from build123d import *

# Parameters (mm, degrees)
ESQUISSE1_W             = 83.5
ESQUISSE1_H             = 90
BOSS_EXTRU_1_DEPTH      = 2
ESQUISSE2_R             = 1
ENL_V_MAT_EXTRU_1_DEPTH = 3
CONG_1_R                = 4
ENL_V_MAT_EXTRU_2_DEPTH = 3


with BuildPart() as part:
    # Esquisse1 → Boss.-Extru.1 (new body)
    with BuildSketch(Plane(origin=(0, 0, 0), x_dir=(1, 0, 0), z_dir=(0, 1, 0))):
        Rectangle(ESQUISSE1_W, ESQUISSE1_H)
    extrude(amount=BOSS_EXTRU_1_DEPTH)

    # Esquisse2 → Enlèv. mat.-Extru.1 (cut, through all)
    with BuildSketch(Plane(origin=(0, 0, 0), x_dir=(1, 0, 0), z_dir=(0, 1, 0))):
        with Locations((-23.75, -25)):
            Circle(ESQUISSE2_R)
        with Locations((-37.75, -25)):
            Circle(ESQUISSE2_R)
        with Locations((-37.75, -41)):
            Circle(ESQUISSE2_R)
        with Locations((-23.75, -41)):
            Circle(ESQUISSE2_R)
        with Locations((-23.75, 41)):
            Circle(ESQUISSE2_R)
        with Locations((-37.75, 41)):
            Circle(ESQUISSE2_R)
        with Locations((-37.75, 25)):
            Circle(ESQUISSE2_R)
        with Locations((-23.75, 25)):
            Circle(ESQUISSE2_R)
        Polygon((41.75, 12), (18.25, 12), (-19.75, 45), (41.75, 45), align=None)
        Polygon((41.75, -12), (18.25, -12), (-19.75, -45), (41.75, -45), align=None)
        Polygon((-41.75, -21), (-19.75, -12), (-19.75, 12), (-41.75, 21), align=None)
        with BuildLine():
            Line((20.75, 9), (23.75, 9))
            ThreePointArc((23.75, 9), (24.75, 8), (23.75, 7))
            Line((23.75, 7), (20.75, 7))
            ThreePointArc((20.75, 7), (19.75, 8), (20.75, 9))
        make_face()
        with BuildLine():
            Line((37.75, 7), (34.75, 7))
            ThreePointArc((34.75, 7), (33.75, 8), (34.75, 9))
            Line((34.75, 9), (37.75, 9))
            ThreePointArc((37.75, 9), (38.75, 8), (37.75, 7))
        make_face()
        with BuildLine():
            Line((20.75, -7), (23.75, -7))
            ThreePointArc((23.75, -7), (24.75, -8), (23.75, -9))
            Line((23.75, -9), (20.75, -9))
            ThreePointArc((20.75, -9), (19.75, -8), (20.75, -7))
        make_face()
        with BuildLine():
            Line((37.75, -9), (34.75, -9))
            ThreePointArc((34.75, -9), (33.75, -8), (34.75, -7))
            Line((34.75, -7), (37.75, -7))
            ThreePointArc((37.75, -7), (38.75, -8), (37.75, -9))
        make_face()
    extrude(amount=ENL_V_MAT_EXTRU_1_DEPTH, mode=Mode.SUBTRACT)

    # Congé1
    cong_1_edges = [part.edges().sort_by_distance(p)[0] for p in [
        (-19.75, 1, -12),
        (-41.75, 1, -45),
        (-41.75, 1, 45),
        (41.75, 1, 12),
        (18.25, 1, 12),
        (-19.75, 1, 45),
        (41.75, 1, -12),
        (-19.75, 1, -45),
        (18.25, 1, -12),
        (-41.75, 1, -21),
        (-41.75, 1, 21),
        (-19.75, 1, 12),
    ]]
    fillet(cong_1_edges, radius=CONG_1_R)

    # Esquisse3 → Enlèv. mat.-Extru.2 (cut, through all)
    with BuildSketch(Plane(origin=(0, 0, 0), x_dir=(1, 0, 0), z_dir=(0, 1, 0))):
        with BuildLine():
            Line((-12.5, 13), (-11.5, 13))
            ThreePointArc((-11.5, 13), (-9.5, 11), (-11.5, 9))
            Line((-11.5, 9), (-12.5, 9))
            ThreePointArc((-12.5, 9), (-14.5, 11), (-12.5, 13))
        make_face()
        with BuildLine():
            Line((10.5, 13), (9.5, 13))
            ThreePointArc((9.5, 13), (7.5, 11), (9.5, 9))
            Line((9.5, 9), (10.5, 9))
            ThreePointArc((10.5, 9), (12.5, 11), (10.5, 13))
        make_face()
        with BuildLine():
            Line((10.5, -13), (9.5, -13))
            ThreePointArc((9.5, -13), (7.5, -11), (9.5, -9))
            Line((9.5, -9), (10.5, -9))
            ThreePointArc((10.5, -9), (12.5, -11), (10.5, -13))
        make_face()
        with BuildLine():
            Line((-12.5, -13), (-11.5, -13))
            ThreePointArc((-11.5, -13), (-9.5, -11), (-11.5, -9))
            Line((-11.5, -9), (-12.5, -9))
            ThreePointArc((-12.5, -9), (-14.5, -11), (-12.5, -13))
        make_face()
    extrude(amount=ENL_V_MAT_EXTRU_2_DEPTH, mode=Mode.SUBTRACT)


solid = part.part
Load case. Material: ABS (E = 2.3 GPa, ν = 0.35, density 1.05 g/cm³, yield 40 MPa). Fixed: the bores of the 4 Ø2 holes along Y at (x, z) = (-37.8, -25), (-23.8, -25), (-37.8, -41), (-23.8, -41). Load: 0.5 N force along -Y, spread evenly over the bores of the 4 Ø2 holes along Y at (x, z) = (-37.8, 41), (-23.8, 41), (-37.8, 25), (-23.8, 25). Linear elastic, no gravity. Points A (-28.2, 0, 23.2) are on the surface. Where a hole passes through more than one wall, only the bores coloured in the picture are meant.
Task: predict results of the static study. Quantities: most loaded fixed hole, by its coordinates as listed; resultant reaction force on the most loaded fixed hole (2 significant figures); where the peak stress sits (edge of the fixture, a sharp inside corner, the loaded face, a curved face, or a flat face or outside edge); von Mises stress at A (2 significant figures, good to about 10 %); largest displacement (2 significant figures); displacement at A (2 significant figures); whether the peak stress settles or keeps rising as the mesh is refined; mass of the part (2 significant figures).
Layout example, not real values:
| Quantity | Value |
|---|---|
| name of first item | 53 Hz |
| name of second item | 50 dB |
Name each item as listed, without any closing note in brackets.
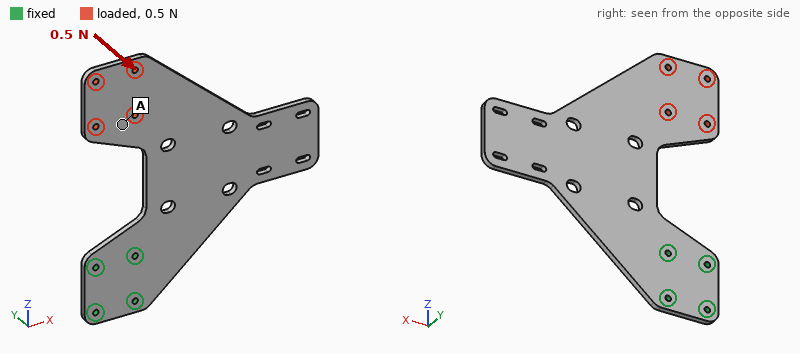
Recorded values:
| Quantity | Value |
|---|---|
| most loaded fixed hole, by its coordinates as listed | (-23.8, -25) |
| resultant reaction force on the most loaded fixed hole | 1.6 N |
| where the peak stress sits | edge of the fixture |
| von Mises stress at A | 0.26 MPa |
| largest displacement | 1.4 mm |
| displacement at A | 0.82 mm |
| whether the peak stress settles or keeps rising as the mesh is refined | keeps rising |
| mass of the part | 8.1 g |
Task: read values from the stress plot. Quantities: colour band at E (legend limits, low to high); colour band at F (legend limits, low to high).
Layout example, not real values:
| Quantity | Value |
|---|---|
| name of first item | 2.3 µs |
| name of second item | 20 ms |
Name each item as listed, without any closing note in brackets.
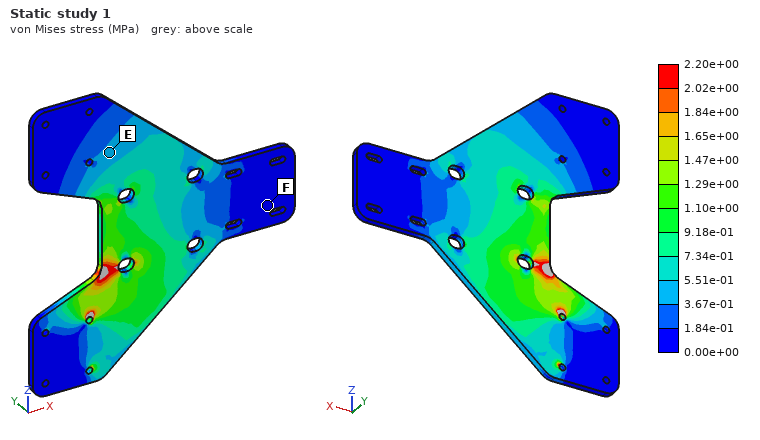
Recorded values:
| Quantity | Value |
|---|---|
| colour band at E | 3.67e-01 to 5.51e-01 MPa |
| colour band at F | 0.00e+00 to 1.84e-01 MPa |
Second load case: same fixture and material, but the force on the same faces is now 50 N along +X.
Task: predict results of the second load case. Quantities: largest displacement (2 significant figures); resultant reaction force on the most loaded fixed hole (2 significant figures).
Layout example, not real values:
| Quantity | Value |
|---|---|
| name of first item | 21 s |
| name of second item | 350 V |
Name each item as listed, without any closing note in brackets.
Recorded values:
| Quantity | Value |
|---|---|
| largest displacement | 1.1 mm |
| resultant reaction force on the most loaded fixed hole | 120 N |
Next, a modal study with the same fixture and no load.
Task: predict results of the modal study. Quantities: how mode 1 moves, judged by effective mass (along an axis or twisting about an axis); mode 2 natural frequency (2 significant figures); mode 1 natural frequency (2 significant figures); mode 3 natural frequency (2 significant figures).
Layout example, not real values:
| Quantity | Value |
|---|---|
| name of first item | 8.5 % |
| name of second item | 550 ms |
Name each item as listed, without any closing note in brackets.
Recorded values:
| Quantity | Value |
|---|---|
| how mode 1 moves, judged by effective mass | along Y |
| mode 2 natural frequency | 100 Hz |
| mode 1 natural frequency | 75 Hz |
| mode 3 natural frequency | 410 Hz |
